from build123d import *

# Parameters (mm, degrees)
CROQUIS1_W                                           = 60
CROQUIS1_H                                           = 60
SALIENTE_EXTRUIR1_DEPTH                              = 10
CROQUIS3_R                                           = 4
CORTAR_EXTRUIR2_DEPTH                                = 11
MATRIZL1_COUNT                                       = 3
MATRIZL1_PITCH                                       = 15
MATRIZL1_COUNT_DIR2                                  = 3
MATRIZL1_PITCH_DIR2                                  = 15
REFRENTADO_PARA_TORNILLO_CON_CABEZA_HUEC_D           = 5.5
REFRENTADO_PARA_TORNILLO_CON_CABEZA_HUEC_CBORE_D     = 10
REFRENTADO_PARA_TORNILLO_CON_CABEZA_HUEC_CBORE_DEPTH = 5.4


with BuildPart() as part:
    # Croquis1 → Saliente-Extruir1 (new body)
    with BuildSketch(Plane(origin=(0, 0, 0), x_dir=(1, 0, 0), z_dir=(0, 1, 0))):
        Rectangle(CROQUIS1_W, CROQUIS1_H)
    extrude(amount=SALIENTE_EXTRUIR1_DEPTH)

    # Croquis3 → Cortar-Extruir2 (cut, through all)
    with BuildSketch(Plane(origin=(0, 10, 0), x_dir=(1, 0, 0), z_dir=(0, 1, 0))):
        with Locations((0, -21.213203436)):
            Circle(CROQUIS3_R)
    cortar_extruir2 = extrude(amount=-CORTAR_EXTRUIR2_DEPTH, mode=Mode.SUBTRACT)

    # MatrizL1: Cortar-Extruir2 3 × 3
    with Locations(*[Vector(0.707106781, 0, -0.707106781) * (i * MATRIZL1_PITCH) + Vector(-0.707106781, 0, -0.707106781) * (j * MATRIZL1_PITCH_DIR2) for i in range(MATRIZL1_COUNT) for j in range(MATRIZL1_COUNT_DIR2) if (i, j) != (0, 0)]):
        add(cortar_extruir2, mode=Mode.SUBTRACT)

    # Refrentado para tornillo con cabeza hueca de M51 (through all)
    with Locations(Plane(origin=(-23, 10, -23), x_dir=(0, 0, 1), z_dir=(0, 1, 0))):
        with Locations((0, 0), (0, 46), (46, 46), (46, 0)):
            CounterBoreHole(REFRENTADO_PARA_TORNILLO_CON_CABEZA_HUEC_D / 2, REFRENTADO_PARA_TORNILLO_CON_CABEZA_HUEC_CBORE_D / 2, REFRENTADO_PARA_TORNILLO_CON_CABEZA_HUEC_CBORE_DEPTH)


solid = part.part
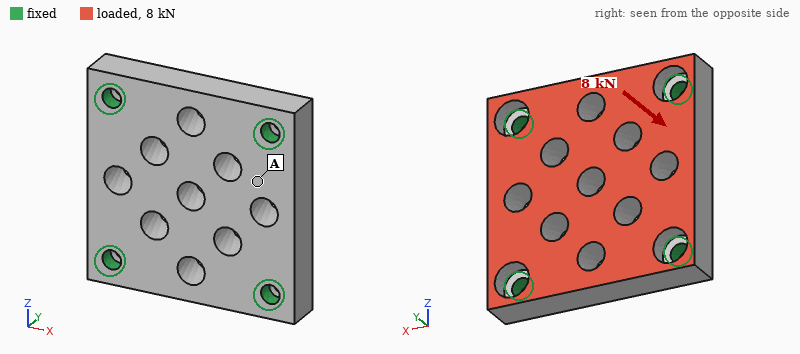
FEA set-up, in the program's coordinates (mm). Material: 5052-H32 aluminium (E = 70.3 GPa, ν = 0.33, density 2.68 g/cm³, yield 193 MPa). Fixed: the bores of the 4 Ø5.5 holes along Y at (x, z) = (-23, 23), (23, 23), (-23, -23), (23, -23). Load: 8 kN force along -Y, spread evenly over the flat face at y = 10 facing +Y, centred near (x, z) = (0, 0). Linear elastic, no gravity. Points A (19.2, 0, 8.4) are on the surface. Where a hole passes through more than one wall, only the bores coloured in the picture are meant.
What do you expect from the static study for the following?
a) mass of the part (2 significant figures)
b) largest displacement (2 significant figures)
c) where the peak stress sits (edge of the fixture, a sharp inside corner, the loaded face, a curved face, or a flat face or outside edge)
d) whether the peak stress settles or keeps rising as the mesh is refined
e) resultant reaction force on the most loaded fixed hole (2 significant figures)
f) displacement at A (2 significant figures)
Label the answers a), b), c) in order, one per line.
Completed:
a) 79 g
b) 29 µm
c) edge of the fixture
d) keeps rising
e) 2.3 kN
f) 17 µm
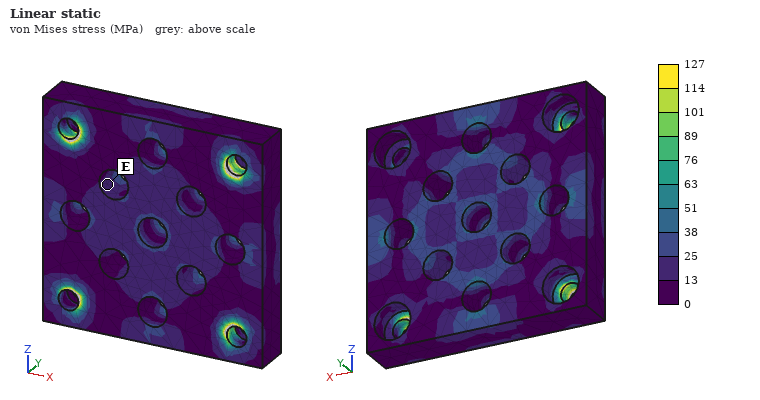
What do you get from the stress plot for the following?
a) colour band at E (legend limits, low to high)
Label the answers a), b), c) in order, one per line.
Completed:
a) 13 to 25 MPa
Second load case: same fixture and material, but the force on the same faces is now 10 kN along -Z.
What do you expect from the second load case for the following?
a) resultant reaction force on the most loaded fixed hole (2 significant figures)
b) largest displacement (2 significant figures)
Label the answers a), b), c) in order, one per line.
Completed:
a) 2.7 kN
b) 15 µm
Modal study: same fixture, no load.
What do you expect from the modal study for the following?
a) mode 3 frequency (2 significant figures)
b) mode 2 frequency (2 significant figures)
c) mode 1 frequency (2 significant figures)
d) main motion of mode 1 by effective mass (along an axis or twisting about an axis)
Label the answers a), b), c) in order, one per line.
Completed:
a) 17 kHz
b) 17 kHz
c) 11 kHz
d) along Y
